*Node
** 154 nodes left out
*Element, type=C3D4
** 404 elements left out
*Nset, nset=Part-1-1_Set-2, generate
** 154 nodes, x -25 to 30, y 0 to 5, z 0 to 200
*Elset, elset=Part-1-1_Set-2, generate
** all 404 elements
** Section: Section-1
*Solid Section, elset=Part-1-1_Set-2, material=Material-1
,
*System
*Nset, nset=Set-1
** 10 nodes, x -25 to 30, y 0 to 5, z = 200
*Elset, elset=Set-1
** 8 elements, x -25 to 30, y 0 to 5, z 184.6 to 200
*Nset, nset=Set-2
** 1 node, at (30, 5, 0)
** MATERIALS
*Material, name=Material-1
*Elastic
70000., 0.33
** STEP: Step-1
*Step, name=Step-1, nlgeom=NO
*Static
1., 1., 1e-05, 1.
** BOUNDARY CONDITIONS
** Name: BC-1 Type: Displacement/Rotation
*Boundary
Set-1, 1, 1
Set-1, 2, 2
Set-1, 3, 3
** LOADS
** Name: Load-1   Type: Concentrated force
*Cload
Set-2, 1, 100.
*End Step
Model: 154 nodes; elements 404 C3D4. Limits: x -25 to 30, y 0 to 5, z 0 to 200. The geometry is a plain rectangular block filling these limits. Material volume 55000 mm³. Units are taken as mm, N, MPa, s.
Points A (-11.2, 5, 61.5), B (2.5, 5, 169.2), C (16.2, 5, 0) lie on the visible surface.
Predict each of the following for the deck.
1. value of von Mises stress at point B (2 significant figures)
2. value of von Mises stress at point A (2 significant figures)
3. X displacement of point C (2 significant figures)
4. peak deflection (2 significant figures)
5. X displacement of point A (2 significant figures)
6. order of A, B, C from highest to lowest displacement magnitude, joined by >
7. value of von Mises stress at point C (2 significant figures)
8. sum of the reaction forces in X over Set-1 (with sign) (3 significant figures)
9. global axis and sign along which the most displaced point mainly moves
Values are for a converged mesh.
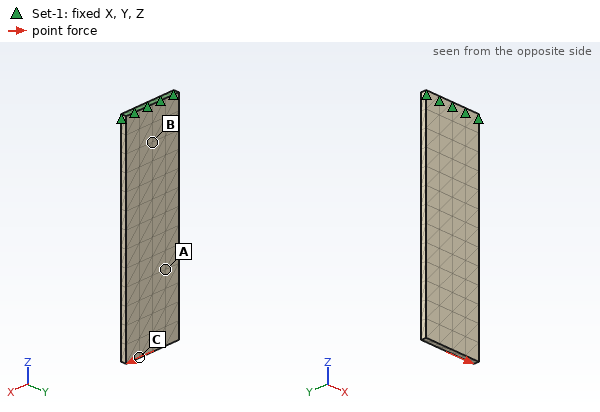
1.9 MPa
2.0 MPa
0.060 mm
0.069 mm
0.034 mm
C > A > B
5.7 MPa
-100 N
+X
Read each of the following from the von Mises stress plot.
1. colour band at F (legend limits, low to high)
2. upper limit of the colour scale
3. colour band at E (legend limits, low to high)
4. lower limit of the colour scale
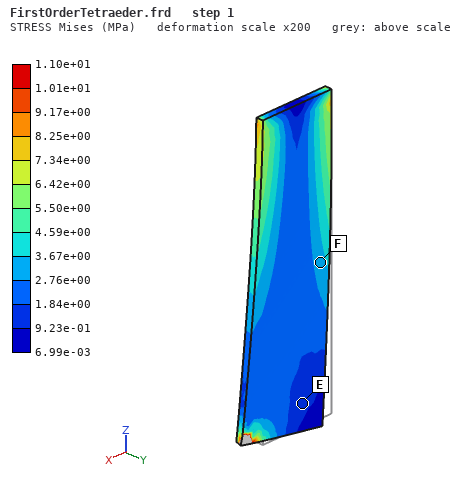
2.76e+00 to 3.67e+00 MPa
1.10e+01 MPa
9.23e-01 to 1.84e+00 MPa
6.99e-03 MPa
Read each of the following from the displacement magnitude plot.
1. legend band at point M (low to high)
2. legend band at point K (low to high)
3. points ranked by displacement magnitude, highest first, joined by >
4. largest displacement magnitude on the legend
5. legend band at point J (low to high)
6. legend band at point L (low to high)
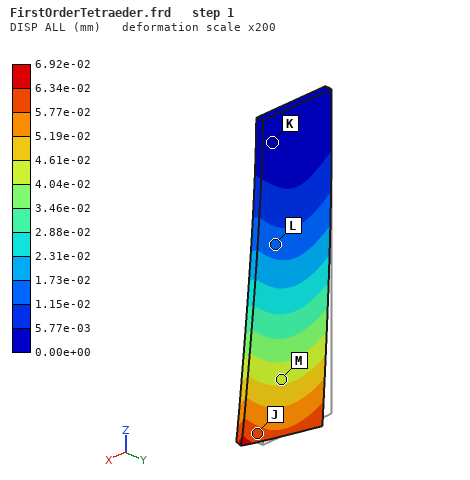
4.04e-02 to 4.61e-02 mm
0.00e+00 to 5.77e-03 mm
J > M > L > K
6.92e-02 mm
5.77e-02 to 6.34e-02 mm
1.15e-02 to 1.73e-02 mm
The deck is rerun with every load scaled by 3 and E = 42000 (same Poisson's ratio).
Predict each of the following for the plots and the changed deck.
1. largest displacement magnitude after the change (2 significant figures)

0.35 mm
